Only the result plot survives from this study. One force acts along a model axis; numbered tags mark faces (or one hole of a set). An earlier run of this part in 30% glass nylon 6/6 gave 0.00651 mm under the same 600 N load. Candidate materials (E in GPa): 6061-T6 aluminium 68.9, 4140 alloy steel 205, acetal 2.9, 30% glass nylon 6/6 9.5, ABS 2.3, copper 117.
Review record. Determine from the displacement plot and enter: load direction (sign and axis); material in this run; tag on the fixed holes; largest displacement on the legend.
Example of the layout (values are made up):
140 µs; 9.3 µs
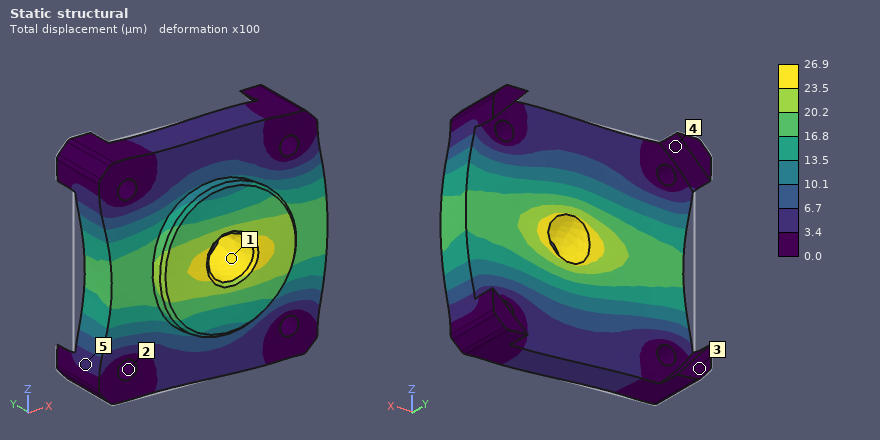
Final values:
+X; ABS; 2; 26.9 µm
